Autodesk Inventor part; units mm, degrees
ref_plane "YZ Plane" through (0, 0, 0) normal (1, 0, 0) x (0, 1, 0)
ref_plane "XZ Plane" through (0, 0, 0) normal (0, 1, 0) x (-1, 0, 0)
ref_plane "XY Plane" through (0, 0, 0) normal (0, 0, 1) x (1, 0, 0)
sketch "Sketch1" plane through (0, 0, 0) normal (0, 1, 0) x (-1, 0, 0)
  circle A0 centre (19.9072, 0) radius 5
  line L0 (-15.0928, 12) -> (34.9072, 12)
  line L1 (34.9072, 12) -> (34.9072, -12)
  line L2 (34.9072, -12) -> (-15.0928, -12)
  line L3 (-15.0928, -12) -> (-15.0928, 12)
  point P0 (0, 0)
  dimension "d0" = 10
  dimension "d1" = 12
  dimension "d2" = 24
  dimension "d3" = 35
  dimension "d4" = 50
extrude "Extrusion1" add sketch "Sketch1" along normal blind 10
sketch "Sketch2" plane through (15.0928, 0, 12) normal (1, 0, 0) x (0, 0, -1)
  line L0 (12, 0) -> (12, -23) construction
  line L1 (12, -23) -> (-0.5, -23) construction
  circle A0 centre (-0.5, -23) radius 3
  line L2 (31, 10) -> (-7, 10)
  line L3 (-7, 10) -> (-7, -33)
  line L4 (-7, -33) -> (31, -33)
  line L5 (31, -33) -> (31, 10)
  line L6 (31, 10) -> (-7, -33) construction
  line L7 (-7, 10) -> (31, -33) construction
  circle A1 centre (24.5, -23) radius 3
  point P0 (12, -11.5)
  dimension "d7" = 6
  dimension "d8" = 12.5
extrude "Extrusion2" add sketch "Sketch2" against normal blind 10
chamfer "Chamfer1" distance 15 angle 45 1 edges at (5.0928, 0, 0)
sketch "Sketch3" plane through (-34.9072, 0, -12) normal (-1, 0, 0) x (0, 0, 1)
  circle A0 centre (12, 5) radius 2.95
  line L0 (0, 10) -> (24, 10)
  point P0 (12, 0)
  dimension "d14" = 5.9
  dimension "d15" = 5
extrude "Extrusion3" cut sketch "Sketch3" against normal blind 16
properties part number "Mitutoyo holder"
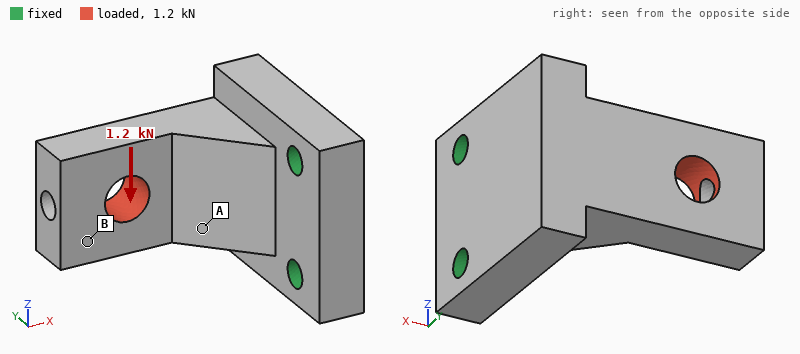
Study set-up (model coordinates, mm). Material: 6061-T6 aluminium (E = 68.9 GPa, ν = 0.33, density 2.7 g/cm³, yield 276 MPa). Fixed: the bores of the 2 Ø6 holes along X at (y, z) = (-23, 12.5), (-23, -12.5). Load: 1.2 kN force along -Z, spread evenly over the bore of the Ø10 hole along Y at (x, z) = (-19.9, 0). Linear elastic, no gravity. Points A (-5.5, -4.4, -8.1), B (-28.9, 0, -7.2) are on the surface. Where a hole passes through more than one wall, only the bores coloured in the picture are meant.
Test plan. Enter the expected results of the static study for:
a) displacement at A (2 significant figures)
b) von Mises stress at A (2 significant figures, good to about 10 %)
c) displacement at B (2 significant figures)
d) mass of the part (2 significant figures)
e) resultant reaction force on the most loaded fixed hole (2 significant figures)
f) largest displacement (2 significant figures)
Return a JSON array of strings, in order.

["19 µm", "18 MPa", "56 µm", "73 g", "1.8 kN", "65 µm"]
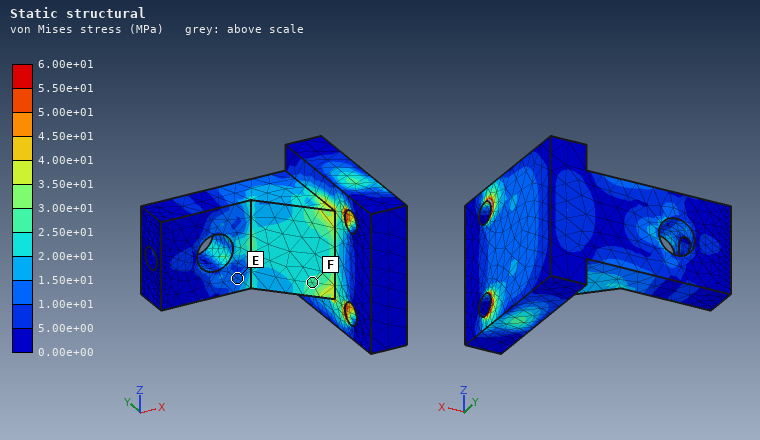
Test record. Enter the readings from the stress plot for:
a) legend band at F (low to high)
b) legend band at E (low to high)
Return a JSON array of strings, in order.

["2.50e+01 to 3.00e+01 MPa", "1.00e+01 to 1.50e+01 MPa"]
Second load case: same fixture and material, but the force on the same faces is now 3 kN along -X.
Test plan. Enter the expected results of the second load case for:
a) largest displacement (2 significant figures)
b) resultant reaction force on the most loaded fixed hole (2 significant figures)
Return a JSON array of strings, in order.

["0.23 mm", "1.5 kN"]
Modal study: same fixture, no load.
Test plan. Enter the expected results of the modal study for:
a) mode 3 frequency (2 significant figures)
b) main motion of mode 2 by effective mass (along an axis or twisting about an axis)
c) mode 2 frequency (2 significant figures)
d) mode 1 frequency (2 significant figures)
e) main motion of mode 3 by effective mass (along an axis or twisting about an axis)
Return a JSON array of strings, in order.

["9200 Hz", "along Z", "5700 Hz", "3200 Hz", "along X"]
